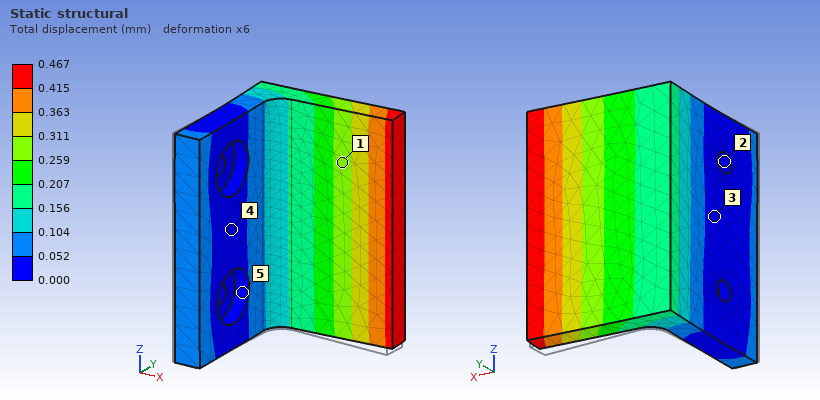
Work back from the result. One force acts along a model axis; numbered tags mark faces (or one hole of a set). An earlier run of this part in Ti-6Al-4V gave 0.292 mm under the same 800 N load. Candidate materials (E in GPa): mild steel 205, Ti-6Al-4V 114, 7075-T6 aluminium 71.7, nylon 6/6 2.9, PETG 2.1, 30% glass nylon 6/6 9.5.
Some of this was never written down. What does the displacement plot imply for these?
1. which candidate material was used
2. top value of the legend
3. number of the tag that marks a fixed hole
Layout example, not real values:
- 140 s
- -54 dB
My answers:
- 7075-T6 aluminium
- 0.467 mm
- 2
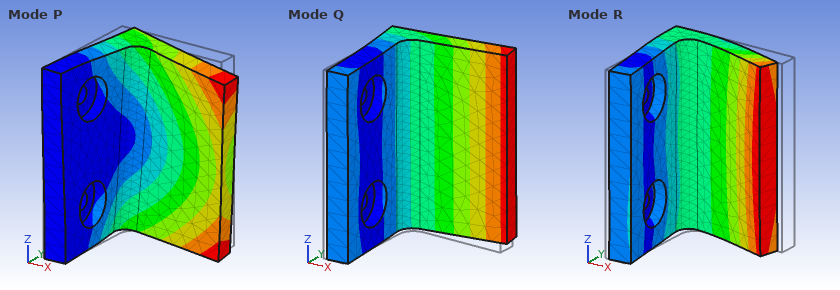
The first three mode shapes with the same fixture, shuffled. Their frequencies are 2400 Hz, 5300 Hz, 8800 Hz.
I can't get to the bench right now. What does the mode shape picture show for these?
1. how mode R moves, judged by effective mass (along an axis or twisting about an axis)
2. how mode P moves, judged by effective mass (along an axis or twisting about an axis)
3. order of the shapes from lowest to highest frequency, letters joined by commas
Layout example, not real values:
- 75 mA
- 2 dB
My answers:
- along X
- along Z
- Q, P, R
